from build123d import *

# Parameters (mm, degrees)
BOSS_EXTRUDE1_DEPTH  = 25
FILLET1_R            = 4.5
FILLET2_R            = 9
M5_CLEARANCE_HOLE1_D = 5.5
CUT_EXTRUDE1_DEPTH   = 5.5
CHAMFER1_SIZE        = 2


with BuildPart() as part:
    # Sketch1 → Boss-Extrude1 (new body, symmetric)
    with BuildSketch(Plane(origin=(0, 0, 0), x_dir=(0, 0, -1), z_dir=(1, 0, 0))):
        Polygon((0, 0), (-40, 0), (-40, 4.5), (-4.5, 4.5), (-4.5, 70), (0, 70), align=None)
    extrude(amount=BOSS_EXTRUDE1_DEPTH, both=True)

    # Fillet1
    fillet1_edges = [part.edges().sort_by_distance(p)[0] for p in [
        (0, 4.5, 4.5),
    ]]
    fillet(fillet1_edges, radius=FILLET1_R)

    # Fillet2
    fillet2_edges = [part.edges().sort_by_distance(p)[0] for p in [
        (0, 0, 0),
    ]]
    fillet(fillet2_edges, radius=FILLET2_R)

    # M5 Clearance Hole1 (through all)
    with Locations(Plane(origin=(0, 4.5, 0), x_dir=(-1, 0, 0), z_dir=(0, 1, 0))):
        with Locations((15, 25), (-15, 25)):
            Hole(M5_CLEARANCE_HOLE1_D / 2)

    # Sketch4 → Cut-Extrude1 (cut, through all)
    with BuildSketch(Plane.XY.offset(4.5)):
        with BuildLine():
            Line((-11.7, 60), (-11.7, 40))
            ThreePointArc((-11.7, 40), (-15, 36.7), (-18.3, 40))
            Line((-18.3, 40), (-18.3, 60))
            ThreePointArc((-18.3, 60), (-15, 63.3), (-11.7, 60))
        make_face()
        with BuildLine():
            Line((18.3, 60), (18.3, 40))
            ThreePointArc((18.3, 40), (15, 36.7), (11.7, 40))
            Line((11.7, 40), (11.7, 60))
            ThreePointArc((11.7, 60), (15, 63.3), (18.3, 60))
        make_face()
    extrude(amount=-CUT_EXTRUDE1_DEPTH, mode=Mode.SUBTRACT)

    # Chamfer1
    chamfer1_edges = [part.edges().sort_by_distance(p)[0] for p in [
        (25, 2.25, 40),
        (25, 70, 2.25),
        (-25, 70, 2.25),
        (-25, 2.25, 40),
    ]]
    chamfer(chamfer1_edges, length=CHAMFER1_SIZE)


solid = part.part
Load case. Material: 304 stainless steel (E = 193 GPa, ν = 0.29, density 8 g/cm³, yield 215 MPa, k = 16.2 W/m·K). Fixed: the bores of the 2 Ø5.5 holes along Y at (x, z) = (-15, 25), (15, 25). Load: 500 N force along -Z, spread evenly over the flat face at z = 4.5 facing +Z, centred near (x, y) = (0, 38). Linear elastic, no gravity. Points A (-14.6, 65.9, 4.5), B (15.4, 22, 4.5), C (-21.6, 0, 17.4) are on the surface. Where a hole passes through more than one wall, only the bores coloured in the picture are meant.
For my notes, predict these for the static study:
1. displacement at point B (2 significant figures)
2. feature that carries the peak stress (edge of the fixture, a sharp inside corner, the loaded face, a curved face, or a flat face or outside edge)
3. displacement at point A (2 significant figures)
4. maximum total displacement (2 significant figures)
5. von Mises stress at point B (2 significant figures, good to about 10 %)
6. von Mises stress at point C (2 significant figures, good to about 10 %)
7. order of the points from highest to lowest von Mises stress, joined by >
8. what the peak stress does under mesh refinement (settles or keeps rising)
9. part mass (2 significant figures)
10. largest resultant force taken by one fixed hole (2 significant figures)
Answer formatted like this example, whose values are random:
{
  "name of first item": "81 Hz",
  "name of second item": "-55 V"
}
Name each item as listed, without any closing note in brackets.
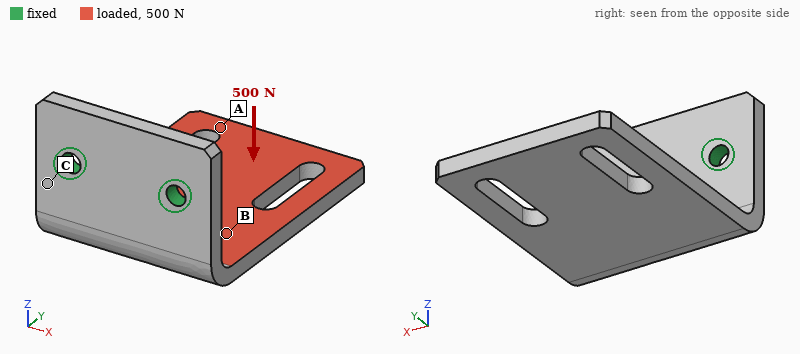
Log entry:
{
  "displacement at point B": "0.13 mm",
  "feature that carries the peak stress": "edge of the fixture",
  "displacement at point A": "0.54 mm",
  "maximum total displacement": "0.59 mm",
  "von Mises stress at point B": "50 MPa",
  "von Mises stress at point C": "100 MPa",
  "order of the points from highest to lowest von Mises stress, joined by >": "C > B > A",
  "what the peak stress does under mesh refinement": "keeps rising",
  "part mass": "170 g",
  "largest resultant force taken by one fixed hole": "270 N"
}
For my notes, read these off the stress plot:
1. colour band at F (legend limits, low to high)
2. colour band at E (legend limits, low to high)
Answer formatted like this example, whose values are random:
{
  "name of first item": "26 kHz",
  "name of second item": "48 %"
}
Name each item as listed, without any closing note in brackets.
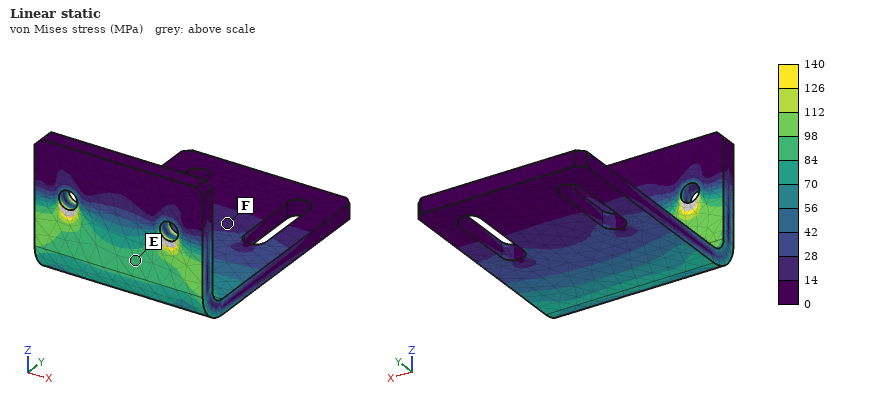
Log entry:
{
  "colour band at F": "14 to 28 MPa",
  "colour band at E": "84 to 98 MPa"
}
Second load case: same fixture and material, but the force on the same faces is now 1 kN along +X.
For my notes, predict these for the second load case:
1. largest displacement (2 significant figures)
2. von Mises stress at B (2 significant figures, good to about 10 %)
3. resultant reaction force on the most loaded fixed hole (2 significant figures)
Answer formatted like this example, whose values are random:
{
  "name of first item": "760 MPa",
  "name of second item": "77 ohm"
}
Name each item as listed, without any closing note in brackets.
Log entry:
{
  "largest displacement": "0.22 mm",
  "von Mises stress at B": "38 MPa",
  "resultant reaction force on the most loaded fixed hole": "1.3 kN"
}
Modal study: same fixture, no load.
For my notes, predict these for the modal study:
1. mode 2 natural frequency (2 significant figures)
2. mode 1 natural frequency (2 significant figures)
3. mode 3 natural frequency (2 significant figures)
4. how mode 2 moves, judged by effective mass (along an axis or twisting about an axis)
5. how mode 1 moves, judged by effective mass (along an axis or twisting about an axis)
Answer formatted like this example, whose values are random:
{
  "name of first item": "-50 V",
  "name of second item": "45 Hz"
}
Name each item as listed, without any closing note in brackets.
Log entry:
{
  "mode 2 natural frequency": "1300 Hz",
  "mode 1 natural frequency": "570 Hz",
  "mode 3 natural frequency": "2400 Hz",
  "how mode 2 moves, judged by effective mass": "along X",
  "how mode 1 moves, judged by effective mass": "along Z"
}
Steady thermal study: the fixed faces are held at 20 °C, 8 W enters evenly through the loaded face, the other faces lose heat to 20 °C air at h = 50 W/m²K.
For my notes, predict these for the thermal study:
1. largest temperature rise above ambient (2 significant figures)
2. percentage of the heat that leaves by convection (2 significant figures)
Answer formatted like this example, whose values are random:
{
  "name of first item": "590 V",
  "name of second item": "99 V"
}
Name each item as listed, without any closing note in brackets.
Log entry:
{
  "largest temperature rise above ambient": "31 K",
  "percentage of the heat that leaves by convection": "80 %"
}
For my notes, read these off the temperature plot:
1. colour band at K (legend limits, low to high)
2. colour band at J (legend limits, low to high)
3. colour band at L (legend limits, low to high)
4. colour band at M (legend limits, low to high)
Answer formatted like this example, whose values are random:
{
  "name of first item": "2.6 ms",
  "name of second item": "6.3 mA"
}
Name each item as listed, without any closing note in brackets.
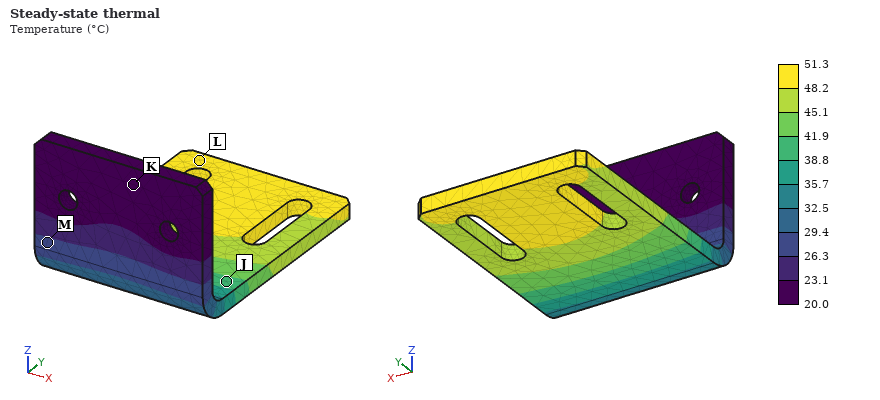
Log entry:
{
  "colour band at K": "20.0 to 23.1 °C",
  "colour band at J": "38.8 to 41.9 °C",
  "colour band at L": "48.2 to 51.3 °C",
  "colour band at M": "26.3 to 29.4 °C"
}
